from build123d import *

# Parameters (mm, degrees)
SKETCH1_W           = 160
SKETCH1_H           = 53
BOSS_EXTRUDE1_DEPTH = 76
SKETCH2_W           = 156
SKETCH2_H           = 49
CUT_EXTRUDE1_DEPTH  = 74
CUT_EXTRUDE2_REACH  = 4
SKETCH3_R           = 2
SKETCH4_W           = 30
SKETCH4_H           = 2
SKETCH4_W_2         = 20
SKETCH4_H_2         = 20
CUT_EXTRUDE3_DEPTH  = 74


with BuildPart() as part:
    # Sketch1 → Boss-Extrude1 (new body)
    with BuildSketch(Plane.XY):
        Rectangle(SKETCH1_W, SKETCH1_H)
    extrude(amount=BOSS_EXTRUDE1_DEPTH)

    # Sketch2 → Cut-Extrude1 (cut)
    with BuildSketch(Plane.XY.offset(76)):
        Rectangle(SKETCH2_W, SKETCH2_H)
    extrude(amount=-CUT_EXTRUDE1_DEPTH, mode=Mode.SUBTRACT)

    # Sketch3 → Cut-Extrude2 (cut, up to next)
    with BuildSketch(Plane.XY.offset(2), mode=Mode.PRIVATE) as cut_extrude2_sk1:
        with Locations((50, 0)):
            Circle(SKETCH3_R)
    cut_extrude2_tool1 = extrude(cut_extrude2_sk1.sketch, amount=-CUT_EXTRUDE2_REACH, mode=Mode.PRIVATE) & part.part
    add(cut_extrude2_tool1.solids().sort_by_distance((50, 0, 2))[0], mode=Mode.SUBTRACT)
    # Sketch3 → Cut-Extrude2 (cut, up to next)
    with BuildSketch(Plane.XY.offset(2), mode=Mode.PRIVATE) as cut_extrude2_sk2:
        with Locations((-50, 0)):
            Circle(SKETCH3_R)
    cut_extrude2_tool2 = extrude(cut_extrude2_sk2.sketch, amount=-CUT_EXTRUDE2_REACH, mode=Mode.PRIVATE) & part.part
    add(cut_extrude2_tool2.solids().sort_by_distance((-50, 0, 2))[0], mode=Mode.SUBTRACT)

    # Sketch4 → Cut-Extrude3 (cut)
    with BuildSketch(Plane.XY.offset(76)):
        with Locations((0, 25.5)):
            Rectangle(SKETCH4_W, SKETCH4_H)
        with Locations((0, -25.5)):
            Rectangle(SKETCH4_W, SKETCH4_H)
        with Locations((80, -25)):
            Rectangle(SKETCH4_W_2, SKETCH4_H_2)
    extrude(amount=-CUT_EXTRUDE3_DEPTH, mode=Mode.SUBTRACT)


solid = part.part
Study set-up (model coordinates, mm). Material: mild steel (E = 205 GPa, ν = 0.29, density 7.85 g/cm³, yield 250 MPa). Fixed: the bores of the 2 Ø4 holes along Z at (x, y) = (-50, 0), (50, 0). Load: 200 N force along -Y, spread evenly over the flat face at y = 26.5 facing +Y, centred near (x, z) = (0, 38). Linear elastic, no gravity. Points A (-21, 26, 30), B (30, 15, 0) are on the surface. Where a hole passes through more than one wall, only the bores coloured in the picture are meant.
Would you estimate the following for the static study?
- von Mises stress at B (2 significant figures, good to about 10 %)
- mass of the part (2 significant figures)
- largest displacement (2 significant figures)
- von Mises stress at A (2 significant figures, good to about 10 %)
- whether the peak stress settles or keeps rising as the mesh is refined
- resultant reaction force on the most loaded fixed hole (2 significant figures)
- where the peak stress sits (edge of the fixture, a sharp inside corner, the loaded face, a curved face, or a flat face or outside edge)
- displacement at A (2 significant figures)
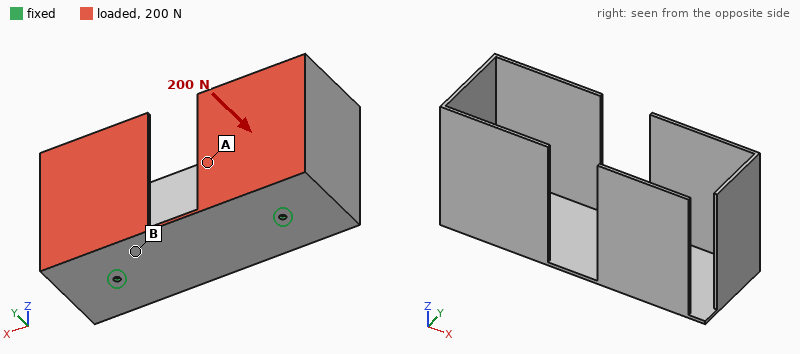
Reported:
37 MPa
530 g
0.68 mm
17 MPa
keeps rising
100 N
edge of the fixture
0.23 mm
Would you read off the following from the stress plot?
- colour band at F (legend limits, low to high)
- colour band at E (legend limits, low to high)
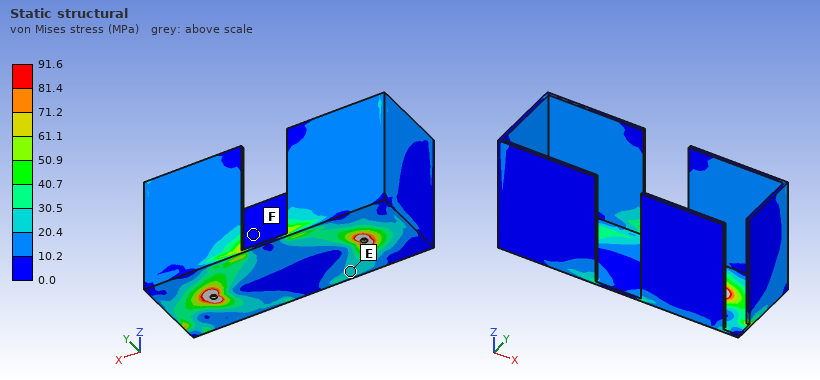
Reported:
0.0 to 10.2 MPa
20.4 to 30.5 MPa
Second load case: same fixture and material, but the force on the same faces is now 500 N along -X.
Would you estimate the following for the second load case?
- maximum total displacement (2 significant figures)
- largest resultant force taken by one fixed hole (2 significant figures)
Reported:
0.58 mm
320 N
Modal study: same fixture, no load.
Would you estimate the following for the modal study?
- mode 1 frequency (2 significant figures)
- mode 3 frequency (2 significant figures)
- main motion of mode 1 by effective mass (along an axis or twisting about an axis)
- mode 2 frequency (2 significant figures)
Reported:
180 Hz
240 Hz
along Y
200 Hz
